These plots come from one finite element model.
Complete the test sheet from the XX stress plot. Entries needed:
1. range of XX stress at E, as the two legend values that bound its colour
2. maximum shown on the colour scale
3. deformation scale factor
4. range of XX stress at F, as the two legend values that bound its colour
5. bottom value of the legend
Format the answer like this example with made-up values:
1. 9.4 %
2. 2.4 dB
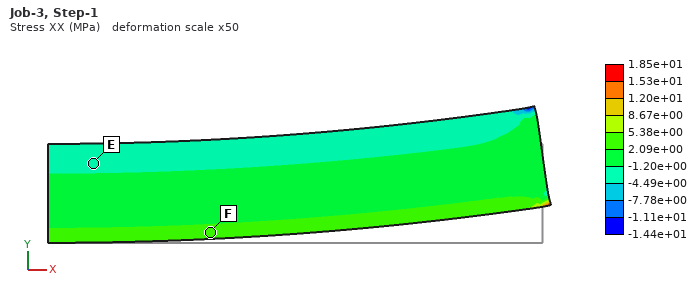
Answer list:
1. -4.49e+00 to -1.20e+00 MPa
2. 1.85e+01 MPa
3. 50
4. 2.09e+00 to 5.38e+00 MPa
5. -1.44e+01 MPa
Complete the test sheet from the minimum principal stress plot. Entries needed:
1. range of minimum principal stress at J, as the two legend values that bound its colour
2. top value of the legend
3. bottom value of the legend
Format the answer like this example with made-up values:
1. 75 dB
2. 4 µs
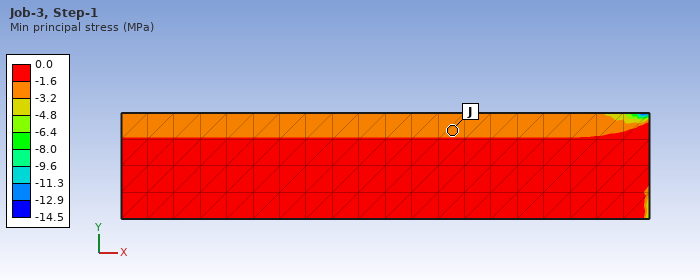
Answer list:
1. -3.2 to -1.6 MPa
2. 0.0 MPa
3. -14.5 MPa
